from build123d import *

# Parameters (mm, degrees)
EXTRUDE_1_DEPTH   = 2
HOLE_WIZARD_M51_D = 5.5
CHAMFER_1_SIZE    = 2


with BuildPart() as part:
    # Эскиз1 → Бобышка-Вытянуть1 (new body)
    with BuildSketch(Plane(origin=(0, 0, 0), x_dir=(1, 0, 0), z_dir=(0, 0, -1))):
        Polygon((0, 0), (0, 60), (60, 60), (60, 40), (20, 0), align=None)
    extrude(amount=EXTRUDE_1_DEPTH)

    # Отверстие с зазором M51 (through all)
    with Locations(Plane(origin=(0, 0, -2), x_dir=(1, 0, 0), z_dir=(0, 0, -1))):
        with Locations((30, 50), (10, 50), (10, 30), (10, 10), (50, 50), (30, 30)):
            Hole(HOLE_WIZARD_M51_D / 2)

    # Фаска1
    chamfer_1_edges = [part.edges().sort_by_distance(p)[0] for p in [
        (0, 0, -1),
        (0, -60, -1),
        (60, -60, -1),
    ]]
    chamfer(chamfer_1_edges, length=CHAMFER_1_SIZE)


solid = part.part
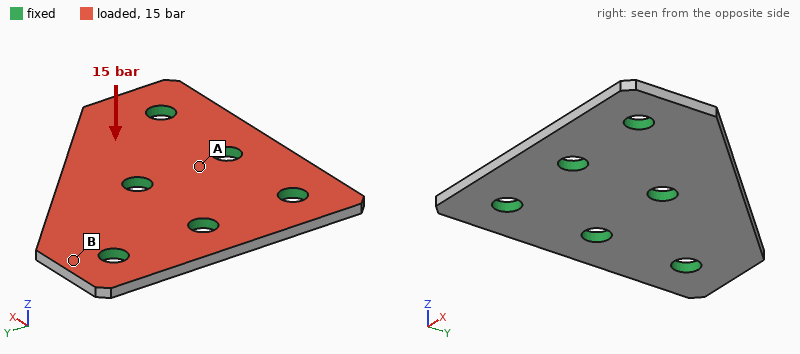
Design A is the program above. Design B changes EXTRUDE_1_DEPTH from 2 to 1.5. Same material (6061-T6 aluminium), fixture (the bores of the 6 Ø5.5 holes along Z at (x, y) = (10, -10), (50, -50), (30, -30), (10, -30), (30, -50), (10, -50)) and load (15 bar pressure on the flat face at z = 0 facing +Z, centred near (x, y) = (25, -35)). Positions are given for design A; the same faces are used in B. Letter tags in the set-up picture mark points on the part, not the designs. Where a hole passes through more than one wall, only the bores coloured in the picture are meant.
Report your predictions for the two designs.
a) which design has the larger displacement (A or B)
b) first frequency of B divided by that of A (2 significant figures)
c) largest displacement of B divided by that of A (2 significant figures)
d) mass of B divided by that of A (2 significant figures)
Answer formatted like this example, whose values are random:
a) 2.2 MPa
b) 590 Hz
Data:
a) B
b) 0.76
c) 2.3
d) 0.75
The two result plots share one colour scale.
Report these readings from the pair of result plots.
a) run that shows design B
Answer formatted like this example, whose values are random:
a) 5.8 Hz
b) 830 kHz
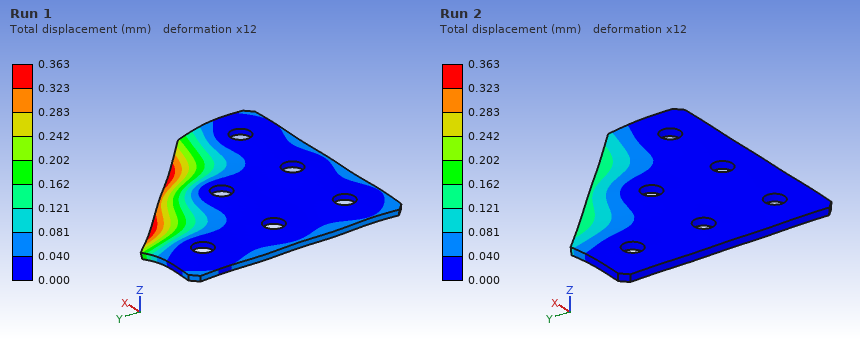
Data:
a) Run 1
